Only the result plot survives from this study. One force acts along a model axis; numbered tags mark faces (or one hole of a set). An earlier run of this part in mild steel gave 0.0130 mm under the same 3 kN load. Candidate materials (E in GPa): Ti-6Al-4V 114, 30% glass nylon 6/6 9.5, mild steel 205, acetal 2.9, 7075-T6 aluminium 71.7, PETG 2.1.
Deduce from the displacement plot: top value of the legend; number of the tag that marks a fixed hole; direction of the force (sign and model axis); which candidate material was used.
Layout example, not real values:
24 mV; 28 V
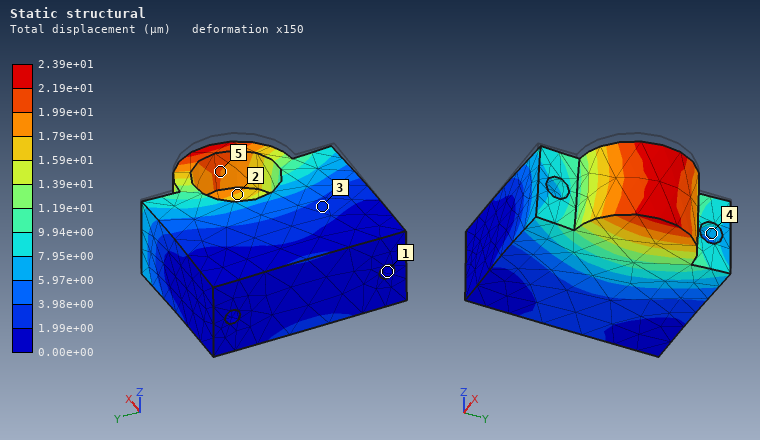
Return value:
2.39e+01 µm; 1; -Z; Ti-6Al-4V
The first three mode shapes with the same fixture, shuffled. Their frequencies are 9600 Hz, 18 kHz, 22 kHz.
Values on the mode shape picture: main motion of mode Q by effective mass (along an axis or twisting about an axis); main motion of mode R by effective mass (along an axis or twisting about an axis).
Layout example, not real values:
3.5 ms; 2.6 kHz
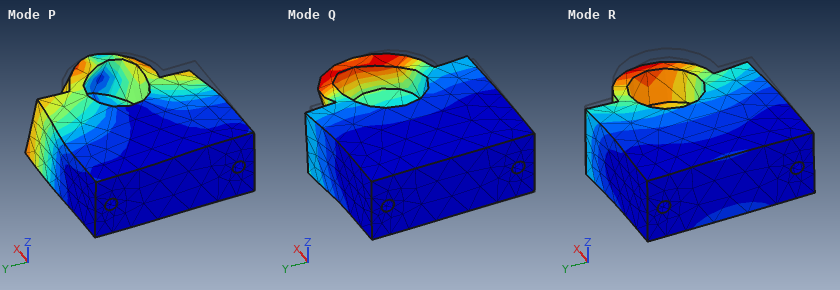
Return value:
along Y; along Z
